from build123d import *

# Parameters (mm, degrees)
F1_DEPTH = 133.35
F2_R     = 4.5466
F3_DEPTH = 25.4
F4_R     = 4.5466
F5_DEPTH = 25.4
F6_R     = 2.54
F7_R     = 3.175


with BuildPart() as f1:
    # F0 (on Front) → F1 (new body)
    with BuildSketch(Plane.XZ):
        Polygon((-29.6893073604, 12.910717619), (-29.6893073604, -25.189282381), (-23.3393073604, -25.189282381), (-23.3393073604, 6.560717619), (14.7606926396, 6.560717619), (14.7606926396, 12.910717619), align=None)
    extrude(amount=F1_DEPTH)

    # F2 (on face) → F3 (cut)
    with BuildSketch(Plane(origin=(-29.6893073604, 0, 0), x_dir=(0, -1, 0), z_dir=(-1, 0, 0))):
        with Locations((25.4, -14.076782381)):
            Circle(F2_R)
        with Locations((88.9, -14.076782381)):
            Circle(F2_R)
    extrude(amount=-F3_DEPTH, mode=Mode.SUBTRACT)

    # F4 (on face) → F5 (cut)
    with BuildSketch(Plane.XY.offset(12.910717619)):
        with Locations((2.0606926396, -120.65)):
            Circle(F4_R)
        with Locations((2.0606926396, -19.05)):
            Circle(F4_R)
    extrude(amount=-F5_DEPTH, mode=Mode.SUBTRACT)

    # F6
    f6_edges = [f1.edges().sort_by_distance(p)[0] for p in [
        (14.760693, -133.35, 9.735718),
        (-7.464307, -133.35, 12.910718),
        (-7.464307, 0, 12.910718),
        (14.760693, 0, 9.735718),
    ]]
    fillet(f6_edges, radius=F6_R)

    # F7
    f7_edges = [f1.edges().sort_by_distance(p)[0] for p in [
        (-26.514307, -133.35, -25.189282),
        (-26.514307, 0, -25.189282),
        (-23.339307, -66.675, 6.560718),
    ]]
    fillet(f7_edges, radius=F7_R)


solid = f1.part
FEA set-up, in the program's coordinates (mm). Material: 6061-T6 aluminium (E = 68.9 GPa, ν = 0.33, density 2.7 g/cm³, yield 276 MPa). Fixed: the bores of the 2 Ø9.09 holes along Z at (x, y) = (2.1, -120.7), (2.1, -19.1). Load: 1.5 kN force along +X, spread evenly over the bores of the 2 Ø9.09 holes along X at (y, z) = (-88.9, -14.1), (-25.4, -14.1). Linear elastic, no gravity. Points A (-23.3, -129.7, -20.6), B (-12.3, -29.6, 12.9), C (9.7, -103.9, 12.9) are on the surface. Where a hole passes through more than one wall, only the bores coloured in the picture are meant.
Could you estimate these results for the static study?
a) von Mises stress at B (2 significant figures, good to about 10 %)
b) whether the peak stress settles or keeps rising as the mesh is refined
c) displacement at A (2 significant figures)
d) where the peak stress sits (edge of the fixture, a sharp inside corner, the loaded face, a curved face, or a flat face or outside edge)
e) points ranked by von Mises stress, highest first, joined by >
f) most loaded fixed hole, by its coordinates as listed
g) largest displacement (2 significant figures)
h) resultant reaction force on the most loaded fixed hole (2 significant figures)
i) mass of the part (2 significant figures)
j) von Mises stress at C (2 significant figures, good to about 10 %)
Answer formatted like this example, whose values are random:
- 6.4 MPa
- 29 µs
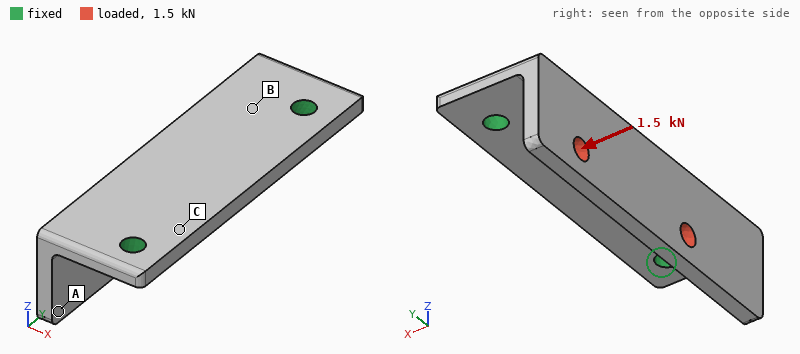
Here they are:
- 42 MPa
- keeps rising
- 0.17 mm
- edge of the fixture
- B > C > A
- (2.1, -19.1)
- 0.30 mm
- 990 N
- 170 g
- 20 MPa
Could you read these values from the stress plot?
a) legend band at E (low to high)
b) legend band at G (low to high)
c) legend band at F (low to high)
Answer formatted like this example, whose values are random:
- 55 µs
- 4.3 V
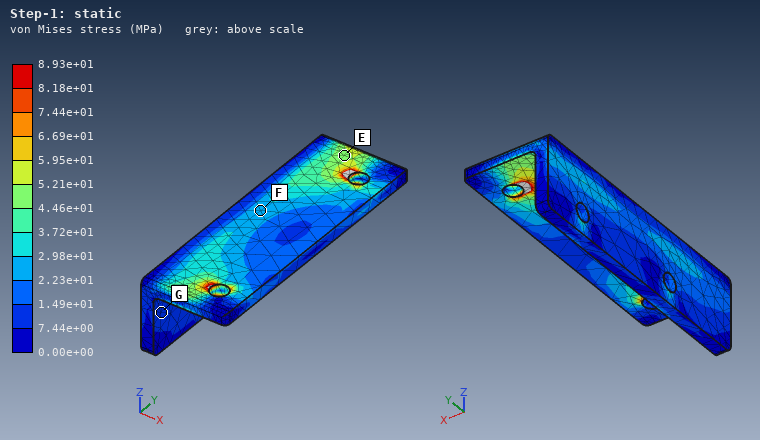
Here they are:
- 4.46e+01 to 5.21e+01 MPa
- 7.44e+00 to 1.49e+01 MPa
- 2.23e+01 to 2.98e+01 MPa
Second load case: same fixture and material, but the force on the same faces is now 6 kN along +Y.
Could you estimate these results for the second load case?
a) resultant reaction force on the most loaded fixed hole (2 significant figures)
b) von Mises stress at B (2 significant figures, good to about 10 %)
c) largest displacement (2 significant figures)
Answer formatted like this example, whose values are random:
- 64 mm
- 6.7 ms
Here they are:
- 3.7 kN
- 29 MPa
- 0.22 mm
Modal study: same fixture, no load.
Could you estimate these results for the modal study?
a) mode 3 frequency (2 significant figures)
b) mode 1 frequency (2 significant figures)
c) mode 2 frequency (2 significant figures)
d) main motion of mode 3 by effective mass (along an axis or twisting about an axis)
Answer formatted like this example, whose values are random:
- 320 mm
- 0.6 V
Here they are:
- 3700 Hz
- 1600 Hz
- 2600 Hz
- along Z
